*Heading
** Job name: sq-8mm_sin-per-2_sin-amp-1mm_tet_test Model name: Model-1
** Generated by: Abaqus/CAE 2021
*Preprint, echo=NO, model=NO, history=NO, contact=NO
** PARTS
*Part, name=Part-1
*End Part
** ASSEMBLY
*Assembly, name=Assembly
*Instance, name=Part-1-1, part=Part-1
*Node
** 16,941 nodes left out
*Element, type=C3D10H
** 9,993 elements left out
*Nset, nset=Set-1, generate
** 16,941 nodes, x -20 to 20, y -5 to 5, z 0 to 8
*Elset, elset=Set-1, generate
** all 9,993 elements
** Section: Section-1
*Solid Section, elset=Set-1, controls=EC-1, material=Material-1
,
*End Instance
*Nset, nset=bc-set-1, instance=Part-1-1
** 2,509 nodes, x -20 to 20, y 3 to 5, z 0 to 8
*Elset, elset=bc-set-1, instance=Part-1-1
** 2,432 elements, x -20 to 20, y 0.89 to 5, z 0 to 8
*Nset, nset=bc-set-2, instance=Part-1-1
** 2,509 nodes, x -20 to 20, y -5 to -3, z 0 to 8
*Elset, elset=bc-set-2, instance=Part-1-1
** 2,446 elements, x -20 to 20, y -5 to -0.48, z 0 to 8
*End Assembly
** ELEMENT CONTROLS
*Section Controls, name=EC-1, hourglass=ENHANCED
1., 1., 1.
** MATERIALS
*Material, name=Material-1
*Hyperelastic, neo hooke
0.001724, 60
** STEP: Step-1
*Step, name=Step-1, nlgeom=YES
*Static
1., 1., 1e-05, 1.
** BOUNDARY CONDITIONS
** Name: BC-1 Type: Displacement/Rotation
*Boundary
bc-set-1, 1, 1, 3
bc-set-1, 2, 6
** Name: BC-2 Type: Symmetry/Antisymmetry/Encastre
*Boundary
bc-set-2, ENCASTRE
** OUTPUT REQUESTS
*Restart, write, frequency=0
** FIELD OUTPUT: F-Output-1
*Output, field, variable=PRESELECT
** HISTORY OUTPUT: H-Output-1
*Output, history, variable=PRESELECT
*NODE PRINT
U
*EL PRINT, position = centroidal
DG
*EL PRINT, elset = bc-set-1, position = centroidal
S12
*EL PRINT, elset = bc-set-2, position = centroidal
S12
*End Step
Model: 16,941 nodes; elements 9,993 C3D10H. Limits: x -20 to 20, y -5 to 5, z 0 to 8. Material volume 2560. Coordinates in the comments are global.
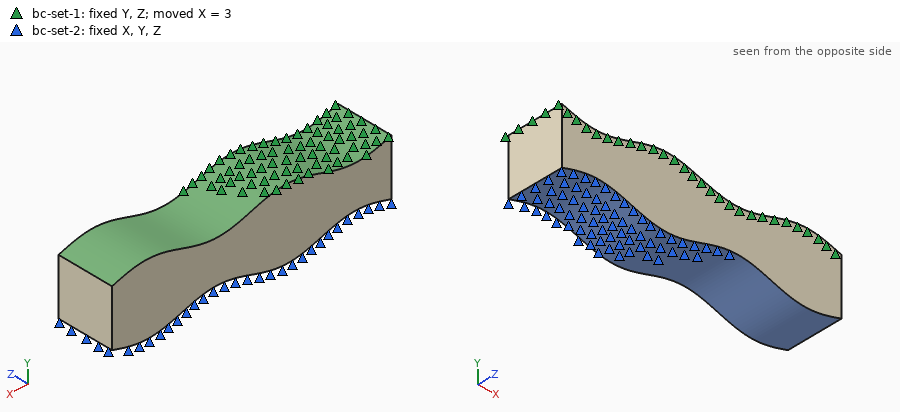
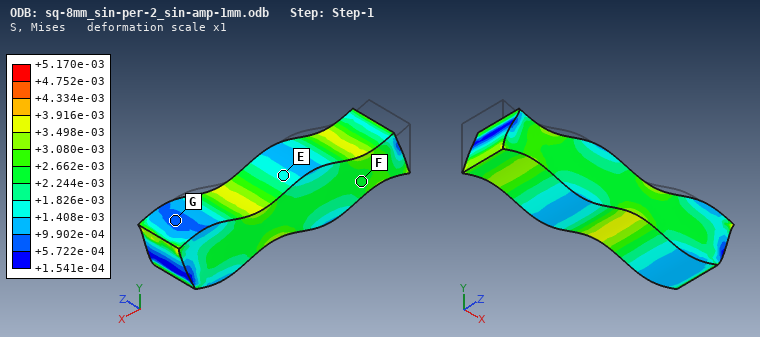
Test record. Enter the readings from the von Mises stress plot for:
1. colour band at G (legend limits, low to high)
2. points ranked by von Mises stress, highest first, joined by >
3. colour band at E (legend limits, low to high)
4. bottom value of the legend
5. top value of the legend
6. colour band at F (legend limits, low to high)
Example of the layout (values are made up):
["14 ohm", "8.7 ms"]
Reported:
["+5.722e-04 to +9.902e-04", "F > E > G", "+1.408e-03 to +1.826e-03", "+1.541e-04", "+5.170e-03", "+2.244e-03 to +2.662e-03"]
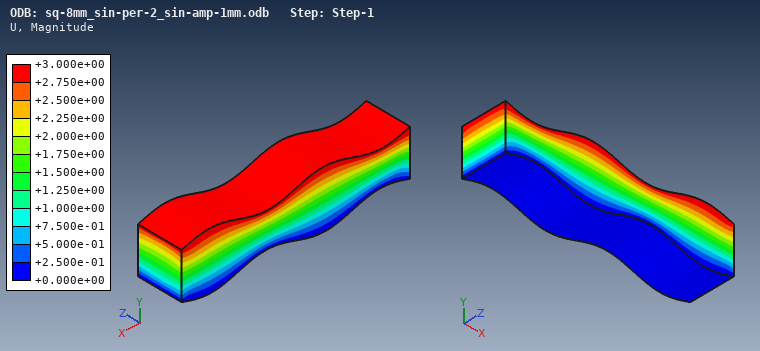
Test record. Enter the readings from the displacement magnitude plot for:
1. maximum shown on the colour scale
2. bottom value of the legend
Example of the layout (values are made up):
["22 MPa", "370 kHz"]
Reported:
["+3.000e+00", "+0.000e+00"]
